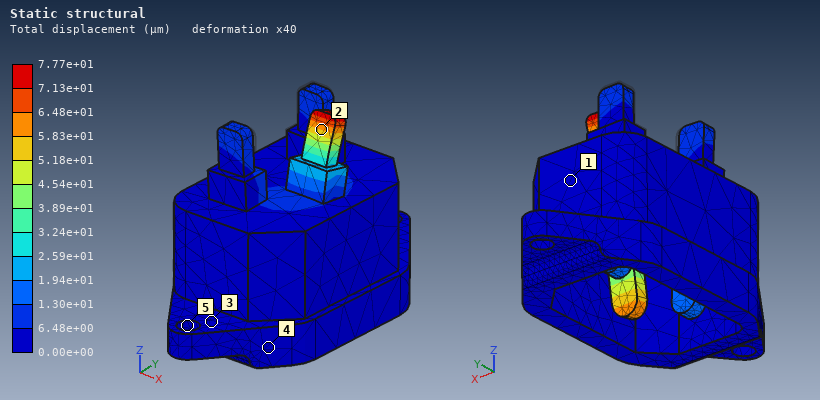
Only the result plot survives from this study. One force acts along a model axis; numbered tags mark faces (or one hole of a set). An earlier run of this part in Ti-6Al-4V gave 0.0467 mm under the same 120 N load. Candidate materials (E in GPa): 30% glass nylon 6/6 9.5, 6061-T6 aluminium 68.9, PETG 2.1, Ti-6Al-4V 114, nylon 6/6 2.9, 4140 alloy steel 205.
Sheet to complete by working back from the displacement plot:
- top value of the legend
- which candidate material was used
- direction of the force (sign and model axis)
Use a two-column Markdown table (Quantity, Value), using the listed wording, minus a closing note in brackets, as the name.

| Quantity | Value |
|---|---|
| top value of the legend | 7.77e+01 µm |
| which candidate material was used | 6061-T6 aluminium |
| direction of the force | +Y |
